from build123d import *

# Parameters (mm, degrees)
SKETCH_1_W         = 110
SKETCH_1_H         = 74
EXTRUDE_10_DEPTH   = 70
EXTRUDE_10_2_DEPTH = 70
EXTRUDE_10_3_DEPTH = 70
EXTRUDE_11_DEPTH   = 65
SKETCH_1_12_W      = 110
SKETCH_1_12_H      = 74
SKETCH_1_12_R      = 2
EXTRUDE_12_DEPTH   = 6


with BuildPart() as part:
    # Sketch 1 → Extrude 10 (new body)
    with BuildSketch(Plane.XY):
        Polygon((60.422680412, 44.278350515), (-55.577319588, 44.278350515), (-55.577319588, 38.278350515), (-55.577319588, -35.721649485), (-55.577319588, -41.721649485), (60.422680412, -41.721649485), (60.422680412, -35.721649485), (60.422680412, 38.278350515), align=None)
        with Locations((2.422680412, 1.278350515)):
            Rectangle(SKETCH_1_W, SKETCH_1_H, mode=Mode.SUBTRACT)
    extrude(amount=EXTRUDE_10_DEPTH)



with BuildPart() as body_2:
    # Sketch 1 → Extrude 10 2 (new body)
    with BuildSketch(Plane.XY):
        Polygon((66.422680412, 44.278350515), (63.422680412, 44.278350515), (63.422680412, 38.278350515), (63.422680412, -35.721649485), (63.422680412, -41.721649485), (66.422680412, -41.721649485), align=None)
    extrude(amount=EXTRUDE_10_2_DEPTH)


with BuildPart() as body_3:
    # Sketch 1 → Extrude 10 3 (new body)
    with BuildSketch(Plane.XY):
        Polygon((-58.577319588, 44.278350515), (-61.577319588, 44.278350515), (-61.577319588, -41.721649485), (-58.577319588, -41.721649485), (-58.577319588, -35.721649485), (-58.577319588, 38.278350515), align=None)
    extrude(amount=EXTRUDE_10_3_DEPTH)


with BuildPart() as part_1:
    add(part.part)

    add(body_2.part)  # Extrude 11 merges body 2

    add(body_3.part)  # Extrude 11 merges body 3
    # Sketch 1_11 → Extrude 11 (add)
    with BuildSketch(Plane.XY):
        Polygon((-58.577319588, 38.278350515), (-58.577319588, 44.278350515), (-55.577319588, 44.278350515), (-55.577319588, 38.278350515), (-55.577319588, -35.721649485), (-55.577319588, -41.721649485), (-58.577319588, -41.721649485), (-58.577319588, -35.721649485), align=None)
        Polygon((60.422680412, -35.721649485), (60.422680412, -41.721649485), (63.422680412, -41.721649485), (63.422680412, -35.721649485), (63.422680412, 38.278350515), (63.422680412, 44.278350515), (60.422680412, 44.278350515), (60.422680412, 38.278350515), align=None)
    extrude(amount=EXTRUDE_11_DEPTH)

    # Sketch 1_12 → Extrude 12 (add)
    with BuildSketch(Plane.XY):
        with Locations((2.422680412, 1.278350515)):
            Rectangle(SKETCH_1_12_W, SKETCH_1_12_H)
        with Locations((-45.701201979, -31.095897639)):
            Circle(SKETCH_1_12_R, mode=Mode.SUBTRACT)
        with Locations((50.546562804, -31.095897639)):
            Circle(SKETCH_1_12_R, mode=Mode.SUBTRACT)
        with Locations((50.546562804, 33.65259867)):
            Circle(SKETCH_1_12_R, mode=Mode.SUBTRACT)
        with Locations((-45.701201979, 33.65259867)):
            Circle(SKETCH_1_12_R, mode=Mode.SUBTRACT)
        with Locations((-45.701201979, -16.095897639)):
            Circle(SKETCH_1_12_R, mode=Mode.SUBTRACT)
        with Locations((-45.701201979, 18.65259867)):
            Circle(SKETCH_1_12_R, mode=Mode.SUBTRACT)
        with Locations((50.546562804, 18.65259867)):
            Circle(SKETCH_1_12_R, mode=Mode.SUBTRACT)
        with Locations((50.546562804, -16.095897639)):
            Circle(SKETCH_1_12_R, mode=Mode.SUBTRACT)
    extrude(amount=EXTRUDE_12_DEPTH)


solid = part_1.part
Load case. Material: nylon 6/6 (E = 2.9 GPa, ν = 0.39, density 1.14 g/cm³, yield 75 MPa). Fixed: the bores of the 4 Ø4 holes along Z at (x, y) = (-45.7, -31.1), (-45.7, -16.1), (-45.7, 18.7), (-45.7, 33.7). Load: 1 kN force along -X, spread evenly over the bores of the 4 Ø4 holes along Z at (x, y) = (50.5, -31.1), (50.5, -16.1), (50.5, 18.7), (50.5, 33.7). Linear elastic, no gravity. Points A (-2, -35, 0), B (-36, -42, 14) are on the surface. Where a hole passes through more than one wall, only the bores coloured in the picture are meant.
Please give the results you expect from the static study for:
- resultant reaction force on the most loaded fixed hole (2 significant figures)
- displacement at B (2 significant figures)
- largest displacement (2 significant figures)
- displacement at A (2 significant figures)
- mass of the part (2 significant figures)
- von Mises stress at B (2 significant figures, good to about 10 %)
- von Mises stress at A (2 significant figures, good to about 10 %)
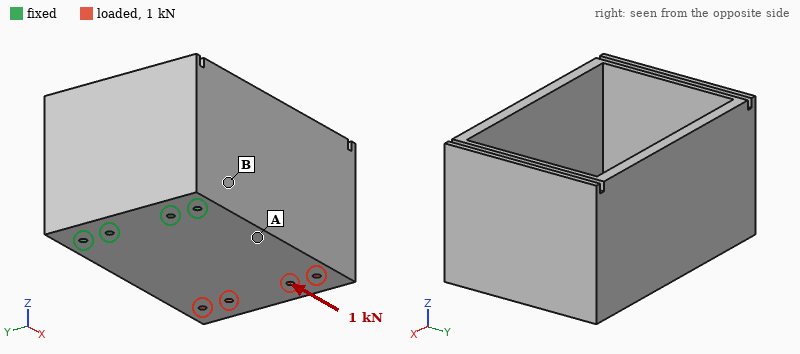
280 N
17 µm
85 µm
32 µm
280 g
0.54 MPa
1.5 MPa
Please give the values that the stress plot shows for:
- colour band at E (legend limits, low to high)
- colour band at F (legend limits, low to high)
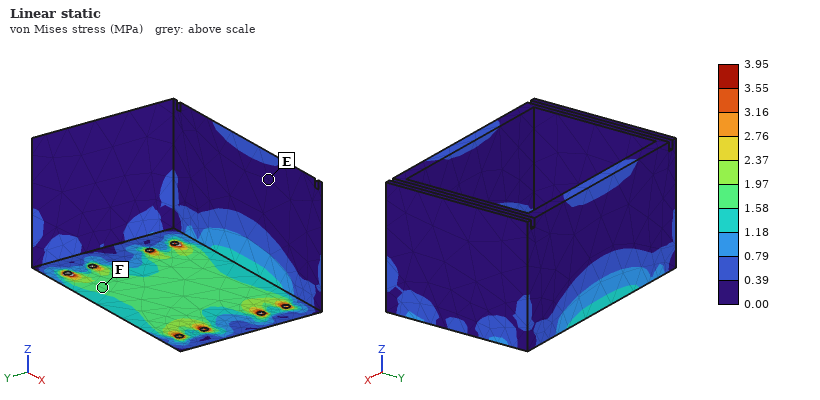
0.00 to 0.39 MPa
1.58 to 1.97 MPa
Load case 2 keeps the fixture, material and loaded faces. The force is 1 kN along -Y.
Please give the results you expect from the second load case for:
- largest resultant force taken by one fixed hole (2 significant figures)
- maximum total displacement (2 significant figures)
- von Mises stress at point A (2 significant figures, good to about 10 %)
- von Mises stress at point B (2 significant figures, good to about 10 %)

1.3 kN
0.57 mm
3.9 MPa
2.8 MPa
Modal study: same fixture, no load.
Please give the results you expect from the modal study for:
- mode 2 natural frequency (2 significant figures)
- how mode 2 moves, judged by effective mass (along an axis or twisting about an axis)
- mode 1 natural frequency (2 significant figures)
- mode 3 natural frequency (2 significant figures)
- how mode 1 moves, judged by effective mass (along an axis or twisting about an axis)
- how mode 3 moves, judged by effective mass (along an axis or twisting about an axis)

270 Hz
along Y
120 Hz
670 Hz
along Z
along Y
